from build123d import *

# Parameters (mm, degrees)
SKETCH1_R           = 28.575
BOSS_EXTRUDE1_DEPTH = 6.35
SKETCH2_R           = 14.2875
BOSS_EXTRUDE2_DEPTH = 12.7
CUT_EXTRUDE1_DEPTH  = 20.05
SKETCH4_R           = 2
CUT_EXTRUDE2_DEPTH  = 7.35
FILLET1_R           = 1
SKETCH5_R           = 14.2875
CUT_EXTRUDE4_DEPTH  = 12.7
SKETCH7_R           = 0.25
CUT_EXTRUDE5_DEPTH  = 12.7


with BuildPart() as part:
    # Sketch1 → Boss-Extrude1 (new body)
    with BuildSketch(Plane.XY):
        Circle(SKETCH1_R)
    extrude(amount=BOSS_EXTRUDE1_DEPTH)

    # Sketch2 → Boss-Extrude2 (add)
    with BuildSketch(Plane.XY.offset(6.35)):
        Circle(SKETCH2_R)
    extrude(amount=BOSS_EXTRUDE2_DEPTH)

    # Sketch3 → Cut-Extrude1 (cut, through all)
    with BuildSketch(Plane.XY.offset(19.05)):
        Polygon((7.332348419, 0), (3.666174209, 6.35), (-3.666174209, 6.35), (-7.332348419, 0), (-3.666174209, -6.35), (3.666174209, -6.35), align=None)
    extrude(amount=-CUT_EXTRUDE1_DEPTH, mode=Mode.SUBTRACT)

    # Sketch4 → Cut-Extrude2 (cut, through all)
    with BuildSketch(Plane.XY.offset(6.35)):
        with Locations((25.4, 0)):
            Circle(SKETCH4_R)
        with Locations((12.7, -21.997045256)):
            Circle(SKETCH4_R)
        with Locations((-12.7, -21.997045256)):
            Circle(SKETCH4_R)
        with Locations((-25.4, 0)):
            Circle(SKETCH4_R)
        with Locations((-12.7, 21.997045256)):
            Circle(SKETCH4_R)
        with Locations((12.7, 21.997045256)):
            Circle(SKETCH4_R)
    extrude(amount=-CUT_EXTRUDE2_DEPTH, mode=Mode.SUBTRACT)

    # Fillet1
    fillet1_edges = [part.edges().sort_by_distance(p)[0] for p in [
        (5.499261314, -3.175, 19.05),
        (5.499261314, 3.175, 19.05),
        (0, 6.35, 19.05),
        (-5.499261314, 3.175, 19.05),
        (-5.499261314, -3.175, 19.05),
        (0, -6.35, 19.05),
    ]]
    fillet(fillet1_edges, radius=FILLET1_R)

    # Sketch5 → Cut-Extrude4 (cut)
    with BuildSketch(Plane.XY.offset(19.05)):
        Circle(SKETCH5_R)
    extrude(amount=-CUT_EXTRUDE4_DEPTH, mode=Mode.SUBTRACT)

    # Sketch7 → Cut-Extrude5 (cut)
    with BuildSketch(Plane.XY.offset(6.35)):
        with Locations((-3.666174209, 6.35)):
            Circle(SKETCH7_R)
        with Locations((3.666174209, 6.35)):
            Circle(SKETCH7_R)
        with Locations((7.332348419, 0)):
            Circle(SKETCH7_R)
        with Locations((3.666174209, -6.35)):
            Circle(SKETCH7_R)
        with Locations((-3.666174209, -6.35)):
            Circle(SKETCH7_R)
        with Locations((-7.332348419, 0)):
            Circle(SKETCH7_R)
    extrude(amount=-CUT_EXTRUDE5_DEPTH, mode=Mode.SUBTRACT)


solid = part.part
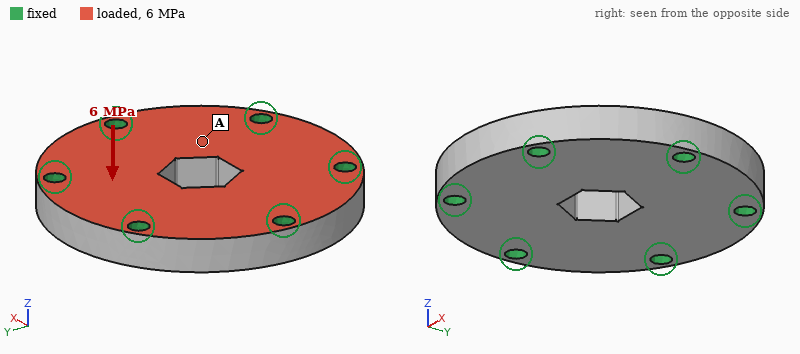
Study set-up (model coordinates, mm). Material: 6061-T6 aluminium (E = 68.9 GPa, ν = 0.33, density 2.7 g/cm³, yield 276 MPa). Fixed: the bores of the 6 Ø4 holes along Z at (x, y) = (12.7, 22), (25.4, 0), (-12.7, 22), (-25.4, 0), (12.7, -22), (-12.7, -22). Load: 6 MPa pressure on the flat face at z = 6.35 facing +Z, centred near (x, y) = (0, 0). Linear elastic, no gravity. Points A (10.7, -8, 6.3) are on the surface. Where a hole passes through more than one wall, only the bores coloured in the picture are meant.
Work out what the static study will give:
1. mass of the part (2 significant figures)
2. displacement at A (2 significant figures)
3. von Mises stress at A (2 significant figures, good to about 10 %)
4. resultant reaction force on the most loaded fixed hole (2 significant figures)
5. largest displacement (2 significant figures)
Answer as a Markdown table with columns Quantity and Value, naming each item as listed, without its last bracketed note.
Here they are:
| Quantity | Value |
|---|---|
| mass of the part | 40 g |
| displacement at A | 25 µm |
| von Mises stress at A | 33 MPa |
| resultant reaction force on the most loaded fixed hole | 2.4 kN |
| largest displacement | 39 µm |
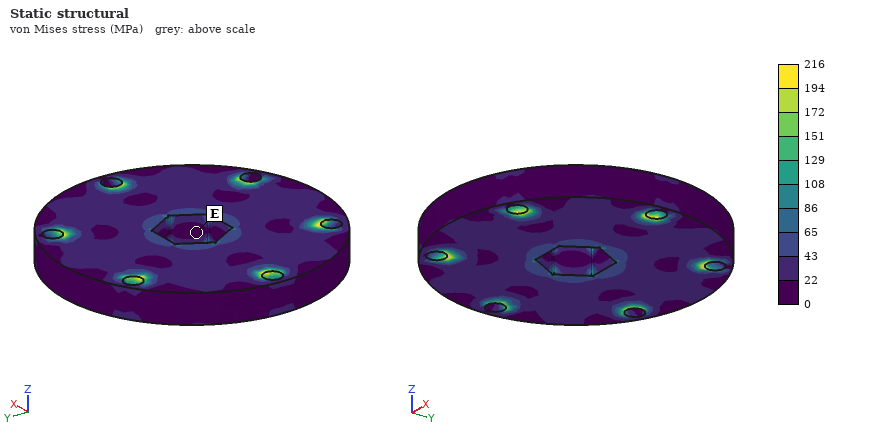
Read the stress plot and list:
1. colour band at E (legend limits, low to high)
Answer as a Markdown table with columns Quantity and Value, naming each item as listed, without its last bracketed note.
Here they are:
| Quantity | Value |
|---|---|
| colour band at E | 0 to 22 MPa |
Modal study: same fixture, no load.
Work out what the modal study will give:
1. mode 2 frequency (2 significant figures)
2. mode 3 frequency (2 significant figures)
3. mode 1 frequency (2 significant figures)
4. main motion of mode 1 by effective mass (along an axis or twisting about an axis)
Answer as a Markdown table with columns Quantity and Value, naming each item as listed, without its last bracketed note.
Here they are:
| Quantity | Value |
|---|---|
| mode 2 frequency | 31 kHz |
| mode 3 frequency | 31 kHz |
| mode 1 frequency | 19 kHz |
| main motion of mode 1 by effective mass | along Z |
